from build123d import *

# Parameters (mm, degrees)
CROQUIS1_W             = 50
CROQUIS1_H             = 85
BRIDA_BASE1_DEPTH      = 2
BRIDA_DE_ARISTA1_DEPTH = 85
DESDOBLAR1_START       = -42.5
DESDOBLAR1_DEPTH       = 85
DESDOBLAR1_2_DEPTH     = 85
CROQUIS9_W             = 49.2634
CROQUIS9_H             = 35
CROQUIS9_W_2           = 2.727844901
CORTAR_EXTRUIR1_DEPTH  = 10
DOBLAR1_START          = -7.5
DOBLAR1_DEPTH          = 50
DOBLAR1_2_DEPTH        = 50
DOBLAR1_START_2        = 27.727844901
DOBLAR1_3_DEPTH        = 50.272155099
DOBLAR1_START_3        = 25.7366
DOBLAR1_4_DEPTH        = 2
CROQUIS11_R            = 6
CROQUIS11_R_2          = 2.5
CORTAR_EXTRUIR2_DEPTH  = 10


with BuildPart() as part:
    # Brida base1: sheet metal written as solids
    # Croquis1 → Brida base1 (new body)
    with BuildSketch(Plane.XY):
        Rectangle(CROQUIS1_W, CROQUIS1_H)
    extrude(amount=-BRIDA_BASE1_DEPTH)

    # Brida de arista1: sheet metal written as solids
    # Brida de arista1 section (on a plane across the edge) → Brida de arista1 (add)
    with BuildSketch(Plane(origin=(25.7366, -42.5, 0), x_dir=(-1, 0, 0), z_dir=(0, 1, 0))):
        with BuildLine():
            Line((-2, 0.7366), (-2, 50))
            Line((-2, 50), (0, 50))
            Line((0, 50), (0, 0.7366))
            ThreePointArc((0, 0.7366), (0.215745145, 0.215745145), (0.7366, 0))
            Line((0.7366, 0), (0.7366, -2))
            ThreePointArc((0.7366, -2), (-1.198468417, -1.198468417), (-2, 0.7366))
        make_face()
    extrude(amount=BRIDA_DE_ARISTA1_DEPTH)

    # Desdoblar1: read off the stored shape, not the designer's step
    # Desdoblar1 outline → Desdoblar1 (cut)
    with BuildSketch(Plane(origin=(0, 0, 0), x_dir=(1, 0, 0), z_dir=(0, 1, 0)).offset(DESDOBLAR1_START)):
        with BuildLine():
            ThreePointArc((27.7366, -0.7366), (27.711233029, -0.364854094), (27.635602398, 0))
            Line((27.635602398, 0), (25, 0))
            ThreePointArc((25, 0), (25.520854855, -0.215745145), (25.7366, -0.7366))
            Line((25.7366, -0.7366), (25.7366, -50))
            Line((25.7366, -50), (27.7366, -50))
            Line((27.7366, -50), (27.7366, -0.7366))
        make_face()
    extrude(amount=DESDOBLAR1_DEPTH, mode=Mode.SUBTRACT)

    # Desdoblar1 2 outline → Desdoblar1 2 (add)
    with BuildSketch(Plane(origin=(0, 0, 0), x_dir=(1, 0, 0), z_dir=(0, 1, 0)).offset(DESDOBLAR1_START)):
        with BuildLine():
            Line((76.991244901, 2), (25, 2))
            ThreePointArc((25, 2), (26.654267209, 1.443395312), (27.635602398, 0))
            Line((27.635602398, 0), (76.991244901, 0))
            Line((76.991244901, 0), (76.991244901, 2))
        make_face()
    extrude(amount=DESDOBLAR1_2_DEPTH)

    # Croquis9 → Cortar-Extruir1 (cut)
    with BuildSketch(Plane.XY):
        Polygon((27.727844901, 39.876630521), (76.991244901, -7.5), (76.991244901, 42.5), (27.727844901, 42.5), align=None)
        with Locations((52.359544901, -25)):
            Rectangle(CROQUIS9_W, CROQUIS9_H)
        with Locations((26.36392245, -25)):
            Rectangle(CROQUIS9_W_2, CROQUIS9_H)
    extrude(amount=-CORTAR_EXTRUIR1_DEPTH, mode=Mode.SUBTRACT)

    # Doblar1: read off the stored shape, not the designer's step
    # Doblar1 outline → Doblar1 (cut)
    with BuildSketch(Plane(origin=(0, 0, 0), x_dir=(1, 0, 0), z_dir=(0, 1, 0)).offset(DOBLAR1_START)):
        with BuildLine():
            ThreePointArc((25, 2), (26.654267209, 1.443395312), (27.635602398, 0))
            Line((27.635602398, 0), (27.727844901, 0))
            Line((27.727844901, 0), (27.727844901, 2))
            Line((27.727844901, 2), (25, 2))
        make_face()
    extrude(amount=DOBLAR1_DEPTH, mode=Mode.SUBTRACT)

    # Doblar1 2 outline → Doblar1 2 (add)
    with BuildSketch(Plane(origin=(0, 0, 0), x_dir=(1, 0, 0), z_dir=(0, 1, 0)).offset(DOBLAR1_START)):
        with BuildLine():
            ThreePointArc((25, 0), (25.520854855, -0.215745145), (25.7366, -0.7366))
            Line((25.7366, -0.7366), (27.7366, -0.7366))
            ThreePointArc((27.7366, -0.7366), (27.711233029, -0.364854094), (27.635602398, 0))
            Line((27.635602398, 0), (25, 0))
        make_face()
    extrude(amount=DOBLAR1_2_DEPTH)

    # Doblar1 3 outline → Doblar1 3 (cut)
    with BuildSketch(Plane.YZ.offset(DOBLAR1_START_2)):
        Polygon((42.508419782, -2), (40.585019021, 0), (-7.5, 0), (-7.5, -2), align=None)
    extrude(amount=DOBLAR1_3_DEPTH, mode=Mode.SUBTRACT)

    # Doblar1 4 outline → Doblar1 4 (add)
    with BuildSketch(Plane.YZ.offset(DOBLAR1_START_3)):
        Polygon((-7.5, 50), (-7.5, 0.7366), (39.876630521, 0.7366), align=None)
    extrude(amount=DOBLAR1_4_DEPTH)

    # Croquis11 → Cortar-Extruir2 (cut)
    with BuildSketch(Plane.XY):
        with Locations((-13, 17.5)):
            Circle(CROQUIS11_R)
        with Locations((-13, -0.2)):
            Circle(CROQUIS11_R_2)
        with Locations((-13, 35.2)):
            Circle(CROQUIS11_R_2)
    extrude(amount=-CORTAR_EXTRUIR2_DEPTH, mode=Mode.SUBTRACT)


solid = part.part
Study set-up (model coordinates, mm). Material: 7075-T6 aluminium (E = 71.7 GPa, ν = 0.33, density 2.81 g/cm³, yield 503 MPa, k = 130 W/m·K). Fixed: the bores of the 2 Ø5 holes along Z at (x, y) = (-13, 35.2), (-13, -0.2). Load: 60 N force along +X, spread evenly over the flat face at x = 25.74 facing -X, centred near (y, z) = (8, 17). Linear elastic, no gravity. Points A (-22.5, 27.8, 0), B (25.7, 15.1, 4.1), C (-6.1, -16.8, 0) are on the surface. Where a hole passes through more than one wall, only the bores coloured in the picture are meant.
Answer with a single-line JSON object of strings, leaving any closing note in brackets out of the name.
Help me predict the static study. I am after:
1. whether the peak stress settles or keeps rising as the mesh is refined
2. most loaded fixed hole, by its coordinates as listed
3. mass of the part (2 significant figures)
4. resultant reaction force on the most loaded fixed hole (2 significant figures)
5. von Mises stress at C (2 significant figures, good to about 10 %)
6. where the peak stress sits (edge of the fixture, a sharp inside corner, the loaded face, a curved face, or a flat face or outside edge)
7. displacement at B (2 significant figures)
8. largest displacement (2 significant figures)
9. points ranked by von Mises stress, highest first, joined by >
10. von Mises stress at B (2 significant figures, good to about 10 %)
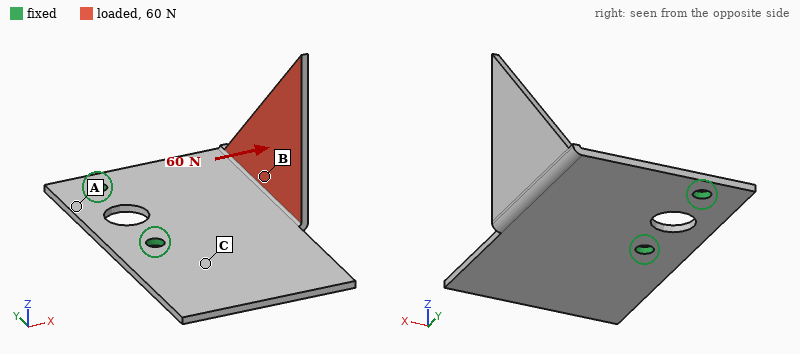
{"whether the peak stress settles or keeps rising as the mesh is refined": "keeps rising", "most loaded fixed hole, by its coordinates as listed": "(-13, -0.2)", "mass of the part": "30 g", "resultant reaction force on the most loaded fixed hole": "46 N", "von Mises stress at C": "15 MPa", "where the peak stress sits": "a sharp inside corner", "displacement at B": "0.26 mm", "largest displacement": "1.1 mm", "points ranked by von Mises stress, highest first, joined by >": "B > C > A", "von Mises stress at B": "27 MPa"}
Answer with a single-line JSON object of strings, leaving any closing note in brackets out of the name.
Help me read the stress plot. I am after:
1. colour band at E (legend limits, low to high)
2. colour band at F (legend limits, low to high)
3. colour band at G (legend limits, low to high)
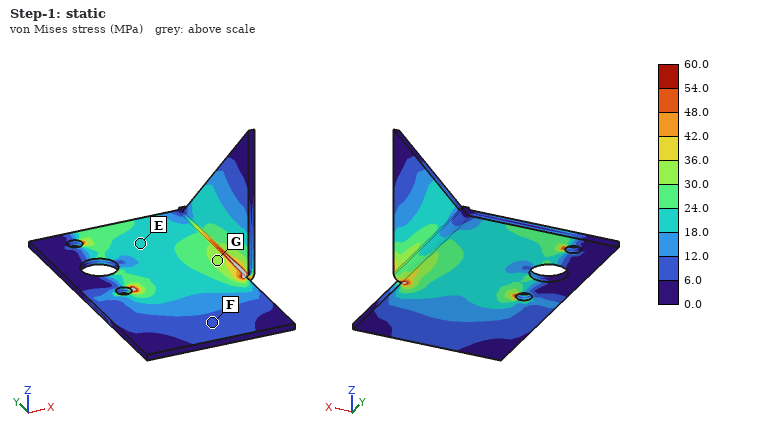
{"colour band at E": "18.0 to 24.0 MPa", "colour band at F": "6.0 to 12.0 MPa", "colour band at G": "30.0 to 36.0 MPa"}
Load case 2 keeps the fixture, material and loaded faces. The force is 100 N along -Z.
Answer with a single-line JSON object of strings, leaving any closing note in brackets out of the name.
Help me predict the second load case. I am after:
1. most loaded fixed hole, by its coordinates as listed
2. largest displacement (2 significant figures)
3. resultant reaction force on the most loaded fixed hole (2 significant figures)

{"most loaded fixed hole, by its coordinates as listed": "(-13, -0.2)", "largest displacement": "1.3 mm", "resultant reaction force on the most loaded fixed hole": "71 N"}
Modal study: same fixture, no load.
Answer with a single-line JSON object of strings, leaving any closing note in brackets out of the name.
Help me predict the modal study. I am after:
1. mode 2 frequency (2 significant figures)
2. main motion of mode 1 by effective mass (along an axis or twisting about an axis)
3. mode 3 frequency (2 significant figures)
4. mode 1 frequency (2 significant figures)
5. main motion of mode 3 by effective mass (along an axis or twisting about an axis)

{"mode 2 frequency": "750 Hz", "main motion of mode 1 by effective mass": "along Z", "mode 3 frequency": "1100 Hz", "mode 1 frequency": "480 Hz", "main motion of mode 3 by effective mass": "along Z"}
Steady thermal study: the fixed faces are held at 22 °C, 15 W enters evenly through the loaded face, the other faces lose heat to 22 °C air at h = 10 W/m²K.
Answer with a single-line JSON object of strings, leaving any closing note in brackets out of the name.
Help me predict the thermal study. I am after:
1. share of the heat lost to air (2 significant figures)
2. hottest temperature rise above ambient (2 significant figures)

{"share of the heat lost to air": "14 %", "hottest temperature rise above ambient": "72 K"}
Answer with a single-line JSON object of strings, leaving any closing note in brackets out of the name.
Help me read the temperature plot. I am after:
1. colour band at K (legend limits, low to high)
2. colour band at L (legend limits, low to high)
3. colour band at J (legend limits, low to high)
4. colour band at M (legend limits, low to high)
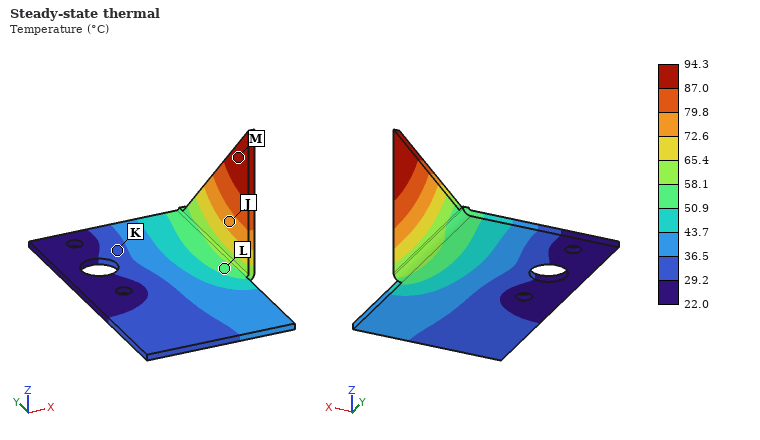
{"colour band at K": "29.2 to 36.5 °C", "colour band at L": "50.9 to 58.1 °C", "colour band at J": "72.6 to 79.8 °C", "colour band at M": "87.0 to 94.3 °C"}
